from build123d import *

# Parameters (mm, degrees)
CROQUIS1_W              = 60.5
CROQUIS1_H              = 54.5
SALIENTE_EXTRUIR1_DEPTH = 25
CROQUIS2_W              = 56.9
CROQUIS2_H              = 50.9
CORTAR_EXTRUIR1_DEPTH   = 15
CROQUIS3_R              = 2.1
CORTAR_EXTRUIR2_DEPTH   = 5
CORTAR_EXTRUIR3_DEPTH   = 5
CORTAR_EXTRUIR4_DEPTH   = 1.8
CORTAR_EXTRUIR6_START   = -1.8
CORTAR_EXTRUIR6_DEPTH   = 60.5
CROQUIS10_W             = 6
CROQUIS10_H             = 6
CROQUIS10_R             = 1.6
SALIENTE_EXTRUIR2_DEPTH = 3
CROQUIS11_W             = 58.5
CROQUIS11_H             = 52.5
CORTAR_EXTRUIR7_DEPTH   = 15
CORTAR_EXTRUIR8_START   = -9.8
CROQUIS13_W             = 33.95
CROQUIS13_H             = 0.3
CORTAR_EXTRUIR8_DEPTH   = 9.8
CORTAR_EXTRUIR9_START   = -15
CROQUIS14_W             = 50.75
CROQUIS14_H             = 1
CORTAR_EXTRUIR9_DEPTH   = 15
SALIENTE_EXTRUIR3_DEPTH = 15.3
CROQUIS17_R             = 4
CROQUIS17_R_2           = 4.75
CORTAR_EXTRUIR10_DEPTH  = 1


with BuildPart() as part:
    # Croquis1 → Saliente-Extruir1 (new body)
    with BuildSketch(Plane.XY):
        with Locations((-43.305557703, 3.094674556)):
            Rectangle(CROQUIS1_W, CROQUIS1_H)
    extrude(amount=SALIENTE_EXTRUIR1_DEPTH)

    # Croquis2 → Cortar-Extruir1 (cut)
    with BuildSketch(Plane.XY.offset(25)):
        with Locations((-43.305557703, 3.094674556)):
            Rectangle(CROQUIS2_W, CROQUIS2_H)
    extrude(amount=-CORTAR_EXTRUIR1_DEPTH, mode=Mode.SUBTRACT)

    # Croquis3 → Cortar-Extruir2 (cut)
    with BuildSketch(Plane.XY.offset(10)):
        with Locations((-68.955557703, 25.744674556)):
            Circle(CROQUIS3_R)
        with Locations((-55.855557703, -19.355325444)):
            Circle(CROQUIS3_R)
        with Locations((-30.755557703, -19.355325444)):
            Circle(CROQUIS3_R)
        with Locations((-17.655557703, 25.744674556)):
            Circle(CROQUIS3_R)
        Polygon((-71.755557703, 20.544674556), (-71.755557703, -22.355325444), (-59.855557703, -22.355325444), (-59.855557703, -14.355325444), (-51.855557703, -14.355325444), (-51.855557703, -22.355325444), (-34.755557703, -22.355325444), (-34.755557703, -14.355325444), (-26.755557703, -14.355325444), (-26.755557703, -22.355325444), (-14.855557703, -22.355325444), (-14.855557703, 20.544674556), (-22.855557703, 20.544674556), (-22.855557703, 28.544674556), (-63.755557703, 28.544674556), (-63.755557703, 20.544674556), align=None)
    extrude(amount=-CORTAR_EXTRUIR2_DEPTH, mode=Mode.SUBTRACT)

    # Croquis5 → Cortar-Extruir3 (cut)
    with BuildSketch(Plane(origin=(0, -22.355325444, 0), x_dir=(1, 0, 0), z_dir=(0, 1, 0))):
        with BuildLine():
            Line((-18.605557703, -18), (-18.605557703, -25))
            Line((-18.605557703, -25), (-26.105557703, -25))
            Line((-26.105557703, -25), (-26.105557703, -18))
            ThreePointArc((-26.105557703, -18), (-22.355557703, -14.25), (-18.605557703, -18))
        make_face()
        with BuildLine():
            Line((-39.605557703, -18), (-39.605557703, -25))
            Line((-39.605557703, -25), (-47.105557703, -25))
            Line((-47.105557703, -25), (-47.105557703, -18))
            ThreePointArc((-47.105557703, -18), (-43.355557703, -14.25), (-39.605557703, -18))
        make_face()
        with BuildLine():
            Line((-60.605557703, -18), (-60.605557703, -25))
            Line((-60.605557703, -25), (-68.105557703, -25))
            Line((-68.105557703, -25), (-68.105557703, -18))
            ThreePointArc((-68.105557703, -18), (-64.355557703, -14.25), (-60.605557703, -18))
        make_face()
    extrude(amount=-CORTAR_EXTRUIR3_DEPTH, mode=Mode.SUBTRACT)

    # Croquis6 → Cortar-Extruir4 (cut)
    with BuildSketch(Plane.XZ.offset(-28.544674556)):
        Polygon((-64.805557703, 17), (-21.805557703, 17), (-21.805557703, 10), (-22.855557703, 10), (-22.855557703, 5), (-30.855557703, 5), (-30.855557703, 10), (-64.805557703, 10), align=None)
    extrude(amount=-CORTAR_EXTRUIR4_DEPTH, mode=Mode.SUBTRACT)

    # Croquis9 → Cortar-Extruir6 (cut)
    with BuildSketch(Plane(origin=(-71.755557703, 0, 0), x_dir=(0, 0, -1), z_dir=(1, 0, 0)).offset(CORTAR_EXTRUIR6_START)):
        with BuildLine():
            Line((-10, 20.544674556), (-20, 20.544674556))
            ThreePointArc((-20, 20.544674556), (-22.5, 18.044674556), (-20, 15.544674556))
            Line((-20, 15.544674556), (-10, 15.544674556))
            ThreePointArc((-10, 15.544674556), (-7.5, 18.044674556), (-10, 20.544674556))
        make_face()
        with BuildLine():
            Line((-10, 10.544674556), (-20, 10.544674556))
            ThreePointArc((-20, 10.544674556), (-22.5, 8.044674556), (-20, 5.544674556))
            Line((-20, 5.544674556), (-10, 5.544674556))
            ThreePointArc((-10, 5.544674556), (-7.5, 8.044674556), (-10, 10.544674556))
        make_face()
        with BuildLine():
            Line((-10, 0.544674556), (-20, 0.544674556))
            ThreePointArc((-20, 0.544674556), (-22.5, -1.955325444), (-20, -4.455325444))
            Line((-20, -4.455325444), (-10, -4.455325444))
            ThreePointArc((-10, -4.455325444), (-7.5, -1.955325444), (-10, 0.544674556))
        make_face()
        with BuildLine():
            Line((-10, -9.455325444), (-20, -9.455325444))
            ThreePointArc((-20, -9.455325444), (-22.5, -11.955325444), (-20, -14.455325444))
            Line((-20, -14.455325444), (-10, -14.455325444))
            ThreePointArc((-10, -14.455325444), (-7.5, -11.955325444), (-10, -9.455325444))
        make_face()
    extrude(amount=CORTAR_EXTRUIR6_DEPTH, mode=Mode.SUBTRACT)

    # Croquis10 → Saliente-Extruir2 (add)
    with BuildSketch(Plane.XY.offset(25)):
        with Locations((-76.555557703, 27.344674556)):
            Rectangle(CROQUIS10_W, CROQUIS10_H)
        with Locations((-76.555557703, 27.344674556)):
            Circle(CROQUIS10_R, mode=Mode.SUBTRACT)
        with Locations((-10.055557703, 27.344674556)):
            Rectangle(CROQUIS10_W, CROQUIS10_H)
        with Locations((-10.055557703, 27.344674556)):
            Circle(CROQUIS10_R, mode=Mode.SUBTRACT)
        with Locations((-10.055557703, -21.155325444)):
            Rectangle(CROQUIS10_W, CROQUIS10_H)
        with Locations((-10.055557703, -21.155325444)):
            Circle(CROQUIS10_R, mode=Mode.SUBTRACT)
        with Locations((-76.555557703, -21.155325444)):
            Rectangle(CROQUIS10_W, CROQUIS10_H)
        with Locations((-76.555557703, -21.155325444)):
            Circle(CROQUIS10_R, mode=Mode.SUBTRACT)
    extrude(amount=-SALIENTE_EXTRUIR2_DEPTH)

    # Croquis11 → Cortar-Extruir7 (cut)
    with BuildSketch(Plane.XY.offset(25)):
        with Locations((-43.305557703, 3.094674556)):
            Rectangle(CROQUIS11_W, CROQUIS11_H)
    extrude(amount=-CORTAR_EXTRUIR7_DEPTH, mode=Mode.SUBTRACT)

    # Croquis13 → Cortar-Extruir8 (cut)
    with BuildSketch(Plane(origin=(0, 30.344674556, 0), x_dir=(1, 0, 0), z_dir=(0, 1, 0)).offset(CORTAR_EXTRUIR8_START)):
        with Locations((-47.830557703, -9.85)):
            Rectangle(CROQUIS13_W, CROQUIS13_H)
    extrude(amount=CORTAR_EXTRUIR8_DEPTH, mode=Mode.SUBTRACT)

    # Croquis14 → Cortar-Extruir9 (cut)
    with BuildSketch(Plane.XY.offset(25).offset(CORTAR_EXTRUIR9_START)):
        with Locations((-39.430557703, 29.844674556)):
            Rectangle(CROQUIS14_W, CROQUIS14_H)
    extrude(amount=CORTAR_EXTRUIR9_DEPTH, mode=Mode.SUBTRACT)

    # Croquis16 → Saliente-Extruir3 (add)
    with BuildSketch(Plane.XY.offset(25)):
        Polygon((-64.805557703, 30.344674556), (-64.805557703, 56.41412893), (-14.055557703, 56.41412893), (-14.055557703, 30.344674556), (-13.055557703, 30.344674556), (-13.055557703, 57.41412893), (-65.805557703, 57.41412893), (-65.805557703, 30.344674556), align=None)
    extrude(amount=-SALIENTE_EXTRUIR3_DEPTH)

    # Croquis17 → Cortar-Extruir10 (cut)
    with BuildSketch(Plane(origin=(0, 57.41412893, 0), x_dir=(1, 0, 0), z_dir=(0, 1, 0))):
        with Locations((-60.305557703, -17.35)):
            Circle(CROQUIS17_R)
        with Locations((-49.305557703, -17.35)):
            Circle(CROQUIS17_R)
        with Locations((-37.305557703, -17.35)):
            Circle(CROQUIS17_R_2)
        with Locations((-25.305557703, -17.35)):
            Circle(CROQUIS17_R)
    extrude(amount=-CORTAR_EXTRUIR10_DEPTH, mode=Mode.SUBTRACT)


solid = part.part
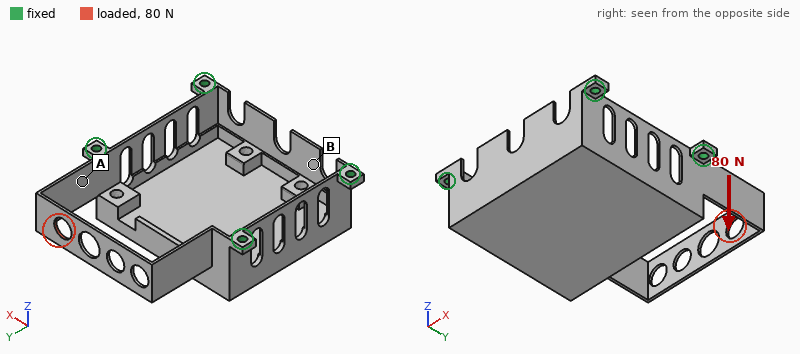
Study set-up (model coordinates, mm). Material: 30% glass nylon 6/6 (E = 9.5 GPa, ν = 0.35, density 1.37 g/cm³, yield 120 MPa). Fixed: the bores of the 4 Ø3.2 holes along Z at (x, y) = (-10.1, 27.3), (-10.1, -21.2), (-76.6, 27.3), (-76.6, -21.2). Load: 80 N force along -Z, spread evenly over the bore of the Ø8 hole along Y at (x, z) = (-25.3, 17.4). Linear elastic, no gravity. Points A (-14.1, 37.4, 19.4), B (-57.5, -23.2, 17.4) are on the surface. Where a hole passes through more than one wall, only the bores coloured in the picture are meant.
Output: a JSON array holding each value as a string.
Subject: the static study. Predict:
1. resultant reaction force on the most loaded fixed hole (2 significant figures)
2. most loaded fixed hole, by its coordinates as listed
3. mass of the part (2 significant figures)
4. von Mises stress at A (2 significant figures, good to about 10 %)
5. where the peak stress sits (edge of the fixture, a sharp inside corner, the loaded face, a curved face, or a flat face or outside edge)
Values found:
["100 N", "(-10.1, 27.3)", "31 g", "14 MPa", "a flat face or outside edge"]
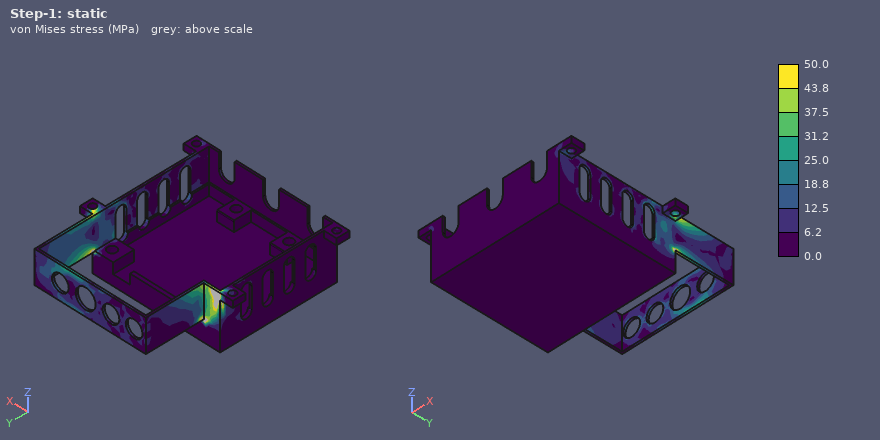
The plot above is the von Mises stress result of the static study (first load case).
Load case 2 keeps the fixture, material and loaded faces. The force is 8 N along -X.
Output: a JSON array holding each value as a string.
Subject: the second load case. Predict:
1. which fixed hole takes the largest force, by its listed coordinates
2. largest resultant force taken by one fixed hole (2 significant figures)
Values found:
["(-10.1, 27.3)", "4.9 N"]
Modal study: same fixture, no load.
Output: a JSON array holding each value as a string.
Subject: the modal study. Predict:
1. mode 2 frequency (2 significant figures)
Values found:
["790 Hz"]
